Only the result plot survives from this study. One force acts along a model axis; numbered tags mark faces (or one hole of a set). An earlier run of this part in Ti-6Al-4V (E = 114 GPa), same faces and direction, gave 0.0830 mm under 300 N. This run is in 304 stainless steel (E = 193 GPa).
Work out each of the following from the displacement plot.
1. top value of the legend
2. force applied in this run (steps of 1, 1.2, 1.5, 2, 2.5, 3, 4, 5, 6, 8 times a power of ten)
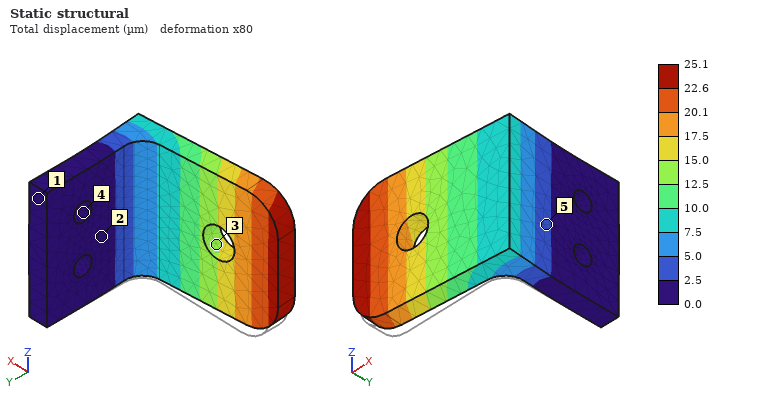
25.1 µm
150 N
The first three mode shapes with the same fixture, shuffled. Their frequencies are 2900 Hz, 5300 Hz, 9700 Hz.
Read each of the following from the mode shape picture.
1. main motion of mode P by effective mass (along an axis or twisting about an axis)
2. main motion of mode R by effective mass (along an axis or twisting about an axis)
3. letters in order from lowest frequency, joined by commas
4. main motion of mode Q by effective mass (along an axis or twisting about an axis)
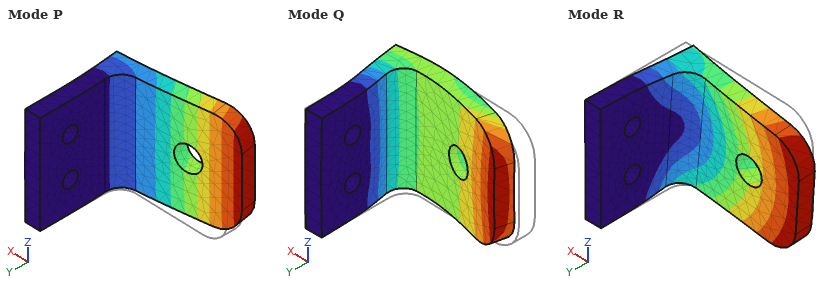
along Y
along Z
P, R, Q
along X
